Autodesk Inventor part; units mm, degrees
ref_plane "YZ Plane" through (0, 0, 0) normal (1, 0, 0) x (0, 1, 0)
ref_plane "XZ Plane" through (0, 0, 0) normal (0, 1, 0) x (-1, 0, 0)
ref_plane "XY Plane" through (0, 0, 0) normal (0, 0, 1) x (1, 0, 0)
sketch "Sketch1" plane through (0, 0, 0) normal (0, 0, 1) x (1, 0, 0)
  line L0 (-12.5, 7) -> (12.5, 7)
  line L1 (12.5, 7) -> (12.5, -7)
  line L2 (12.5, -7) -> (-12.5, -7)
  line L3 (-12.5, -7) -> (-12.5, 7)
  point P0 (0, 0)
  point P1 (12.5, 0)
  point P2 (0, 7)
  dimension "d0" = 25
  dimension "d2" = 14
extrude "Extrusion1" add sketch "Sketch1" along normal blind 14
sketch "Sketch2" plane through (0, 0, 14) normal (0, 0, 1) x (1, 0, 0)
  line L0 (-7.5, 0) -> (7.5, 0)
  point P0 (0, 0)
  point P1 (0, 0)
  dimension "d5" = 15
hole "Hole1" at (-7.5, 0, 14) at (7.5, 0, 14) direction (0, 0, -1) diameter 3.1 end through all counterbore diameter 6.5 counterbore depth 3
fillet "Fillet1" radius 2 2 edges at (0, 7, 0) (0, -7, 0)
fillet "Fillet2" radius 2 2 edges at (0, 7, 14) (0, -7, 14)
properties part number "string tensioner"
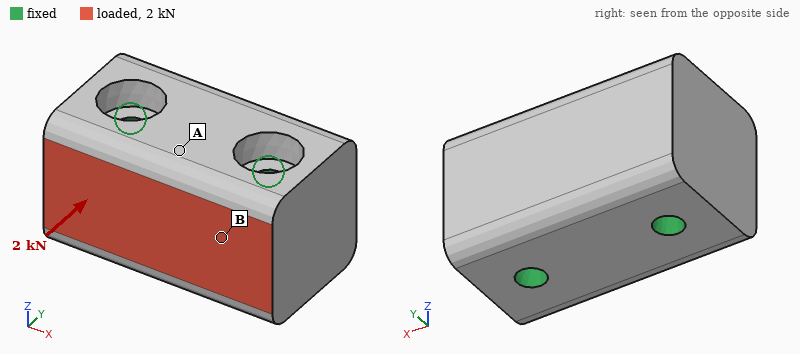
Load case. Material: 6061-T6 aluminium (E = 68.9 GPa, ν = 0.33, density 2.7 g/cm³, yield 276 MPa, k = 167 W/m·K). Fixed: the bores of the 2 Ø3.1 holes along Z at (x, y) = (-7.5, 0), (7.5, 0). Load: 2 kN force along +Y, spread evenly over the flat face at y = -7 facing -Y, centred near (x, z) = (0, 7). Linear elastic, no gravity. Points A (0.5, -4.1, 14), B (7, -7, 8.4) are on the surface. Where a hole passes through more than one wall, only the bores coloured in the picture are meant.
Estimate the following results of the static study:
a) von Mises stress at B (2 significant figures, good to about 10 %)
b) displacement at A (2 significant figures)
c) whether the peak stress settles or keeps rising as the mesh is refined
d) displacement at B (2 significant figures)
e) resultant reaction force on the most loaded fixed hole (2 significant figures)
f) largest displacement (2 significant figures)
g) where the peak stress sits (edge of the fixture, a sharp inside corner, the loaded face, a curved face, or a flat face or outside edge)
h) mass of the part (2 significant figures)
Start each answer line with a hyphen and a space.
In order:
- 9.8 MPa
- 1.3 µm
- keeps rising
- 1.0 µm
- 1.0 kN
- 1.4 µm
- edge of the fixture
- 12 g
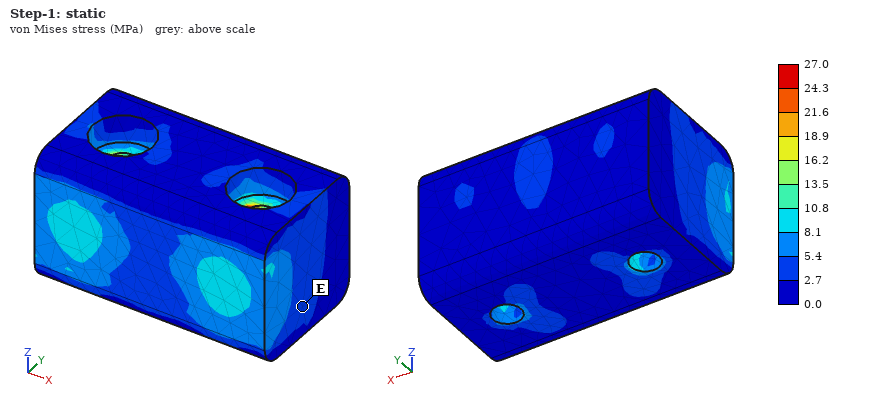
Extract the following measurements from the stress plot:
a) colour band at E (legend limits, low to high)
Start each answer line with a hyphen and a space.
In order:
- 2.7 to 5.4 MPa
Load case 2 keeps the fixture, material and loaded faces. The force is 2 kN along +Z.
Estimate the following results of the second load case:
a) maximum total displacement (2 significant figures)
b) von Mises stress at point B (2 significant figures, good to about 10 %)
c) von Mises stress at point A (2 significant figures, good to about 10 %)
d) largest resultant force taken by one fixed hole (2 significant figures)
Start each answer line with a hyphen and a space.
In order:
- 4.9 µm
- 16 MPa
- 7.2 MPa
- 1.0 kN
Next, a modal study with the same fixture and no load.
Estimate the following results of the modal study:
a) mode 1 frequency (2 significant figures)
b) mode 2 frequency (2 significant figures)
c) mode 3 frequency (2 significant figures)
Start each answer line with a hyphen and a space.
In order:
- 57 kHz
- 72 kHz
- 75 kHz
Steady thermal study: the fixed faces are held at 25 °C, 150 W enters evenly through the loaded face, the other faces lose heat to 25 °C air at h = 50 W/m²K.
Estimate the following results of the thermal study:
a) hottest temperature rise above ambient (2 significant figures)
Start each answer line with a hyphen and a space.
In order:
- 26 K
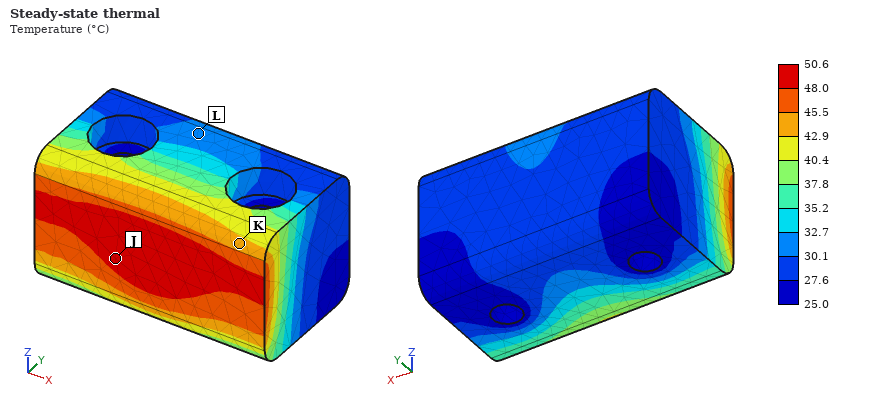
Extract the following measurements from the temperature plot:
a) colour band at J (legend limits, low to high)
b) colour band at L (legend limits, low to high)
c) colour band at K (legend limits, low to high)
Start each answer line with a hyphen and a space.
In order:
- 48.0 to 50.6 °C
- 30.1 to 32.7 °C
- 42.9 to 45.5 °C
